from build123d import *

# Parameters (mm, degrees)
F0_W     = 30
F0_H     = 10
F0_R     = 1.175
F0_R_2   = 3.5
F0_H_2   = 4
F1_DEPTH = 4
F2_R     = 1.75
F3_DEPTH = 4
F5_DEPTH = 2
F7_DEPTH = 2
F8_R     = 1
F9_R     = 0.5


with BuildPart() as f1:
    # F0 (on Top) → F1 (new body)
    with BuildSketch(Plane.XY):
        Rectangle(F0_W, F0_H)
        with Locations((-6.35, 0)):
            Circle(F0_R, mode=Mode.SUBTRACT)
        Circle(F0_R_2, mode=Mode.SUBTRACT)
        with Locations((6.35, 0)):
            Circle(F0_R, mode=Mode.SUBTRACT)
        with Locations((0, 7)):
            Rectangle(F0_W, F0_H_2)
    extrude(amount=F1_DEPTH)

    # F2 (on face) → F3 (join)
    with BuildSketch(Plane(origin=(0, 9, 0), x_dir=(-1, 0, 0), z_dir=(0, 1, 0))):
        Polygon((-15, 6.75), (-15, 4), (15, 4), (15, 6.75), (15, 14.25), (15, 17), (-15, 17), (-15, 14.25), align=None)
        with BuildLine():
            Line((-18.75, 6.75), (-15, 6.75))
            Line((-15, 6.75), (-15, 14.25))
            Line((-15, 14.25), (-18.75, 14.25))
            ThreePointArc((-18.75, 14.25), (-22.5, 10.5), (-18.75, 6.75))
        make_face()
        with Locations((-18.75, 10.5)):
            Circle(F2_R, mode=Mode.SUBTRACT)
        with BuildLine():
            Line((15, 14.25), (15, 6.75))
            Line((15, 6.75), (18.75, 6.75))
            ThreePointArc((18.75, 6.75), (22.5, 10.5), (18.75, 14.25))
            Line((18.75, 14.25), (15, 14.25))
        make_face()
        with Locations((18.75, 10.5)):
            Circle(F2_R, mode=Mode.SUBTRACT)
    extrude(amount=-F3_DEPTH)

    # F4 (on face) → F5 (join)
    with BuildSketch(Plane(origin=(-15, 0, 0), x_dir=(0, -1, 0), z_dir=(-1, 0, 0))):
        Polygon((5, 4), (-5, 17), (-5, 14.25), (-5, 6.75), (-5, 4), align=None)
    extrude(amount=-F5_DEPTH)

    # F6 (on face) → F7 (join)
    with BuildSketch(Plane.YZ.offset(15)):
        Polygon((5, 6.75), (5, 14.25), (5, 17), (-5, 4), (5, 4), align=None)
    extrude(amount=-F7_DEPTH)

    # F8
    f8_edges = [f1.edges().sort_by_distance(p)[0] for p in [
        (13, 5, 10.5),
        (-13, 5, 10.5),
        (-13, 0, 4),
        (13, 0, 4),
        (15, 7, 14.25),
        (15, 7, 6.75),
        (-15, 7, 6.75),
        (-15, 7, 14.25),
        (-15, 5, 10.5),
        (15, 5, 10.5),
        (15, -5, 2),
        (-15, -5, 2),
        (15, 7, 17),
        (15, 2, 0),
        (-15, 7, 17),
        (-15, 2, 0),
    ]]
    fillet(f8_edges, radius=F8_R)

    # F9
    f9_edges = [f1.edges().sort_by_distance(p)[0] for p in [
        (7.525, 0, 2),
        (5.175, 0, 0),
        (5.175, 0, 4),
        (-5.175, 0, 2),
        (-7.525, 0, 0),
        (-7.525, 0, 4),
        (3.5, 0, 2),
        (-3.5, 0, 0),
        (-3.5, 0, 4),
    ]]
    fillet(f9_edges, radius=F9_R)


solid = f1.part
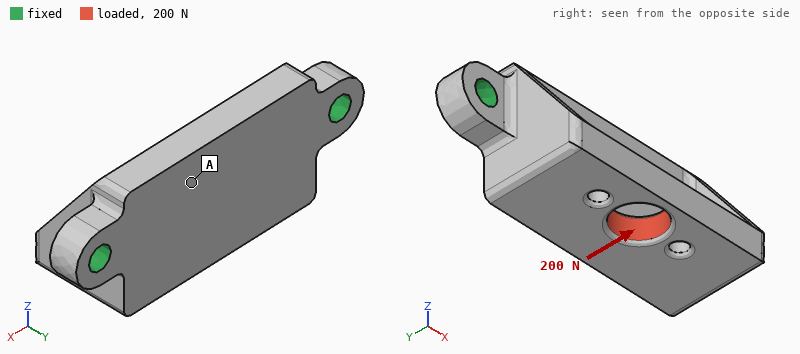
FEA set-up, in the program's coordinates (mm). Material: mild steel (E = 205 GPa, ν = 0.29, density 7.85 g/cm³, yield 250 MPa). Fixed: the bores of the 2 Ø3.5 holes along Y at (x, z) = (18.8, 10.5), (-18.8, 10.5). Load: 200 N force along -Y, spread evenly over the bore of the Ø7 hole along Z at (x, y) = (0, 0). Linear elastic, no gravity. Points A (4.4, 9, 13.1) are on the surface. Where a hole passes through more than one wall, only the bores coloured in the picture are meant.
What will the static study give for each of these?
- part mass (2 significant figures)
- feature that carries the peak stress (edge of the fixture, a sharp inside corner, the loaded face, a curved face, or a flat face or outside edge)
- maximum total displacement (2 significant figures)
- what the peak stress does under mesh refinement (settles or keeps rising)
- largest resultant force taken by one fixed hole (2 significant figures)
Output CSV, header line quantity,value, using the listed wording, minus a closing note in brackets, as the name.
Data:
quantity,value
part mass,29 g
feature that carries the peak stress,edge of the fixture
maximum total displacement,6.9 µm
what the peak stress does under mesh refinement,keeps rising
largest resultant force taken by one fixed hole,100 N
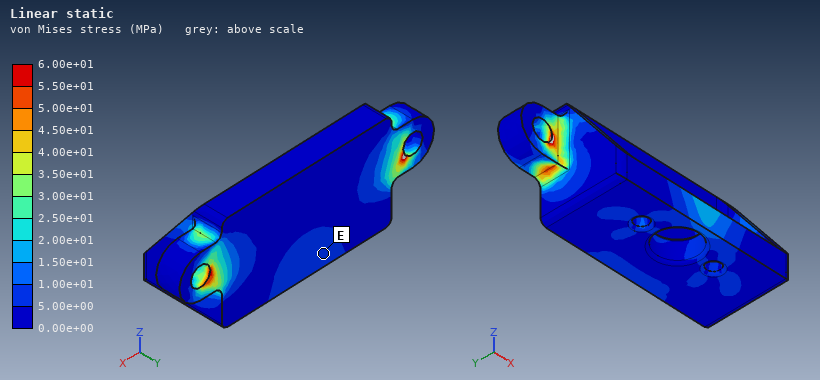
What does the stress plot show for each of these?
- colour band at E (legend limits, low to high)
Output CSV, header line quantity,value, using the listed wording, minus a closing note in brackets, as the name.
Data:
quantity,value
colour band at E,5.00e+00 to 1.00e+01 MPa
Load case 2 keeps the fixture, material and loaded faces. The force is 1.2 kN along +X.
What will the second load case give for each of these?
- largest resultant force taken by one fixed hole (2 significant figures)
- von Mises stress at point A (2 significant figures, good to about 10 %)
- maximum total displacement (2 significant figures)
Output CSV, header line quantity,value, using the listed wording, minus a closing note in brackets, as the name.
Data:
quantity,value
largest resultant force taken by one fixed hole,710 N
von Mises stress at point A,9.3 MPa
maximum total displacement,8.8 µm
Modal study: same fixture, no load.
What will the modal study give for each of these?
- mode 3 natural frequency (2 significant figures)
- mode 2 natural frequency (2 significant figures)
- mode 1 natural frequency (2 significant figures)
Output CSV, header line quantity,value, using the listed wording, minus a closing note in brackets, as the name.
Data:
quantity,value
mode 3 natural frequency,17 kHz
mode 2 natural frequency,16 kHz
mode 1 natural frequency,8300 Hz
